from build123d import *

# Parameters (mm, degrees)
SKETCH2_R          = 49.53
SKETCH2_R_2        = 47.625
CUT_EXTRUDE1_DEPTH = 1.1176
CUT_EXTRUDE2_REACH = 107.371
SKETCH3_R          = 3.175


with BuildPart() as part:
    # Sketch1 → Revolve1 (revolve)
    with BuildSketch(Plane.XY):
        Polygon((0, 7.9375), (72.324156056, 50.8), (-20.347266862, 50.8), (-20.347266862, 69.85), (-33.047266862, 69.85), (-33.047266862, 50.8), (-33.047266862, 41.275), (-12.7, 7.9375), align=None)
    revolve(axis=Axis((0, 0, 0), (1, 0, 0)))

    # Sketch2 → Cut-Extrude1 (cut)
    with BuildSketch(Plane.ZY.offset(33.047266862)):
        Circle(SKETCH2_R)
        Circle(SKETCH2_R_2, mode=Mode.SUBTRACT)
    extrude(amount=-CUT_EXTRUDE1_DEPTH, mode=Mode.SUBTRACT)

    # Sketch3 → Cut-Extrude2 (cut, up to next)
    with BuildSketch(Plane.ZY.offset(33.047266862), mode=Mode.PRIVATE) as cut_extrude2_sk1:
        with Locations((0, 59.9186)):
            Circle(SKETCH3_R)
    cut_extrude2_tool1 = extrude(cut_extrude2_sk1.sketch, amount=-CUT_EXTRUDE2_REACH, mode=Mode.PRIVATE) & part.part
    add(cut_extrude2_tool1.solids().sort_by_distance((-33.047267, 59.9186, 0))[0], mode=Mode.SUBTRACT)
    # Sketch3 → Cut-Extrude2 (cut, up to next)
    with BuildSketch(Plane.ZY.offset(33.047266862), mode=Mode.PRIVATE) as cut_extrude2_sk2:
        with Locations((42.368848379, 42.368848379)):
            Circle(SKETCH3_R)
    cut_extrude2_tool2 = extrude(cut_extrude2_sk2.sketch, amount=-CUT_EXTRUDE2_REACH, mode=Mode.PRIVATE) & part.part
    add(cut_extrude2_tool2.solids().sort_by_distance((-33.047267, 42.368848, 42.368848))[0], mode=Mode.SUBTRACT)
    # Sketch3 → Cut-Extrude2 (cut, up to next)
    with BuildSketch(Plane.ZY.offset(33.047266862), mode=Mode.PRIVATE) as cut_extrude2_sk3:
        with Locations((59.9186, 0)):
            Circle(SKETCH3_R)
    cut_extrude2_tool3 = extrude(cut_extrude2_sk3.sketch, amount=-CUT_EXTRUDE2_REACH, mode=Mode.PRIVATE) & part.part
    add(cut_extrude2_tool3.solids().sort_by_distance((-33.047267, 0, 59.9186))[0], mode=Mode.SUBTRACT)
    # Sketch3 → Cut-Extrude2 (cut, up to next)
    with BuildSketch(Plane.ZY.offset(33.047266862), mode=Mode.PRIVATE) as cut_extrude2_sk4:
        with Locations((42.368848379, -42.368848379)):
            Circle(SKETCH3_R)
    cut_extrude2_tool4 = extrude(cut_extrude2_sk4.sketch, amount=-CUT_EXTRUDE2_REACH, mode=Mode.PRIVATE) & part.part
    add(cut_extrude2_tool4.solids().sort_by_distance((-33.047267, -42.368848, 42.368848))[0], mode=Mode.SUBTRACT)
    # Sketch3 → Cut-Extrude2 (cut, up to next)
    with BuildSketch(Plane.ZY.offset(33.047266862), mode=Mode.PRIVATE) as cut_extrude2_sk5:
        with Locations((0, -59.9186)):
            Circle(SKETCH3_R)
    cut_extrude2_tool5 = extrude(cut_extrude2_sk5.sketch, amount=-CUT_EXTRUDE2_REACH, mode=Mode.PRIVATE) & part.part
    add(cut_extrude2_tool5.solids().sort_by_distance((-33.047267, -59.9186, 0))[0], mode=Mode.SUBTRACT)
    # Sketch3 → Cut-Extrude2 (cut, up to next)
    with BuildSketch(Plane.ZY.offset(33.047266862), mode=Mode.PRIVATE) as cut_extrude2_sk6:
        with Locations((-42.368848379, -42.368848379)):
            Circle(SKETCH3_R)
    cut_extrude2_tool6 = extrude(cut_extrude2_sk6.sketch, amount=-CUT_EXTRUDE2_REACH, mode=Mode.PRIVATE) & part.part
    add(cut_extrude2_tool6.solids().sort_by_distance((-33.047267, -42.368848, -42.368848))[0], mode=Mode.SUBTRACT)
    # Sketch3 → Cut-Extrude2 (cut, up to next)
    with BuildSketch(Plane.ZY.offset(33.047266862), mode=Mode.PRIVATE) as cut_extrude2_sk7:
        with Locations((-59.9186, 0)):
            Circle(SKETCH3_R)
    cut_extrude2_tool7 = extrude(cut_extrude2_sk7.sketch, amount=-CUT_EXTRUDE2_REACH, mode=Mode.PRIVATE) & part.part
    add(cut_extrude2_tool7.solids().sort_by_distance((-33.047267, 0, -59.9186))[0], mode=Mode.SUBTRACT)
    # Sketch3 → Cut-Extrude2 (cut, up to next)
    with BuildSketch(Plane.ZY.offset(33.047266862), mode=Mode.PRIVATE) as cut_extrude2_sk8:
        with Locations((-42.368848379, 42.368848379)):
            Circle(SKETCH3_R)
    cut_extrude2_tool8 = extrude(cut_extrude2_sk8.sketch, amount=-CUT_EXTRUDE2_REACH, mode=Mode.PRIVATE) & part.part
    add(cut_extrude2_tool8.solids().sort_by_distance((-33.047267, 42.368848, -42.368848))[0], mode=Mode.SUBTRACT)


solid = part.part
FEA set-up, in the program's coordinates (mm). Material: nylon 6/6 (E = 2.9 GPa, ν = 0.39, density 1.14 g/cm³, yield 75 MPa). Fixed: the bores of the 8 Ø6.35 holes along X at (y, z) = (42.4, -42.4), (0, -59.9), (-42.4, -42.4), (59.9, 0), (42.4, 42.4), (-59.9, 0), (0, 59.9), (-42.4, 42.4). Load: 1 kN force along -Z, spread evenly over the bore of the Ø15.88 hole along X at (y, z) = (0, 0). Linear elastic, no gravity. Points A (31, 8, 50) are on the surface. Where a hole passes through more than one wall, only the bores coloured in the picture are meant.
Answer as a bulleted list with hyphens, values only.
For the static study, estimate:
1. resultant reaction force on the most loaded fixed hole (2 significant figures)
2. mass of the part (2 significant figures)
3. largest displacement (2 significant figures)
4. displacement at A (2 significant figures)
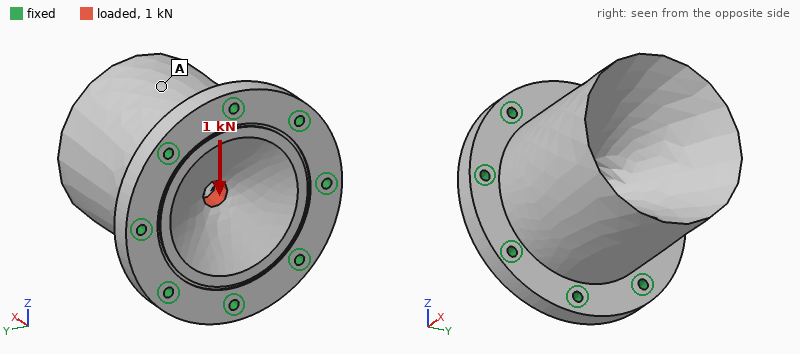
- 210 N
- 760 g
- 14 µm
- 11 µm
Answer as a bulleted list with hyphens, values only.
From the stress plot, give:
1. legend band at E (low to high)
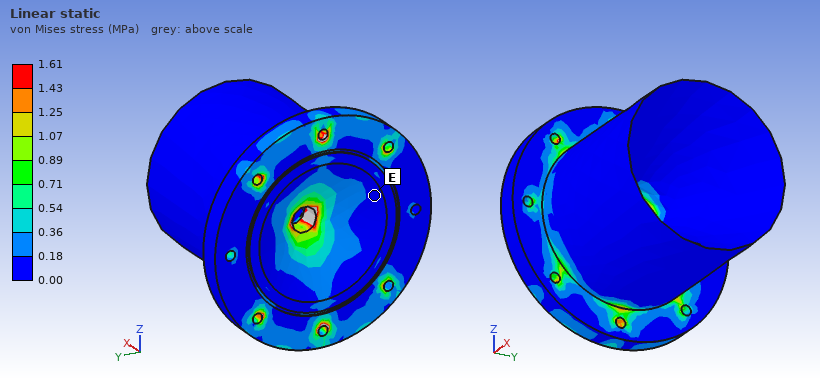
- 0.00 to 0.18 MPa
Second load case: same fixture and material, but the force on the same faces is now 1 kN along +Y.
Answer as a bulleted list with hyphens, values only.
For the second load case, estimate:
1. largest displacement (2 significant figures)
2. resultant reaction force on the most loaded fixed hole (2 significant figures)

- 14 µm
- 210 N
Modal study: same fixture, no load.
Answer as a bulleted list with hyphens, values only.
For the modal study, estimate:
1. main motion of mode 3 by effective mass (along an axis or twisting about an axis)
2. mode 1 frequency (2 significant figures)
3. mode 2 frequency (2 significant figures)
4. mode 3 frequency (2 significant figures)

- along X
- 1400 Hz
- 1400 Hz
- 2000 Hz
